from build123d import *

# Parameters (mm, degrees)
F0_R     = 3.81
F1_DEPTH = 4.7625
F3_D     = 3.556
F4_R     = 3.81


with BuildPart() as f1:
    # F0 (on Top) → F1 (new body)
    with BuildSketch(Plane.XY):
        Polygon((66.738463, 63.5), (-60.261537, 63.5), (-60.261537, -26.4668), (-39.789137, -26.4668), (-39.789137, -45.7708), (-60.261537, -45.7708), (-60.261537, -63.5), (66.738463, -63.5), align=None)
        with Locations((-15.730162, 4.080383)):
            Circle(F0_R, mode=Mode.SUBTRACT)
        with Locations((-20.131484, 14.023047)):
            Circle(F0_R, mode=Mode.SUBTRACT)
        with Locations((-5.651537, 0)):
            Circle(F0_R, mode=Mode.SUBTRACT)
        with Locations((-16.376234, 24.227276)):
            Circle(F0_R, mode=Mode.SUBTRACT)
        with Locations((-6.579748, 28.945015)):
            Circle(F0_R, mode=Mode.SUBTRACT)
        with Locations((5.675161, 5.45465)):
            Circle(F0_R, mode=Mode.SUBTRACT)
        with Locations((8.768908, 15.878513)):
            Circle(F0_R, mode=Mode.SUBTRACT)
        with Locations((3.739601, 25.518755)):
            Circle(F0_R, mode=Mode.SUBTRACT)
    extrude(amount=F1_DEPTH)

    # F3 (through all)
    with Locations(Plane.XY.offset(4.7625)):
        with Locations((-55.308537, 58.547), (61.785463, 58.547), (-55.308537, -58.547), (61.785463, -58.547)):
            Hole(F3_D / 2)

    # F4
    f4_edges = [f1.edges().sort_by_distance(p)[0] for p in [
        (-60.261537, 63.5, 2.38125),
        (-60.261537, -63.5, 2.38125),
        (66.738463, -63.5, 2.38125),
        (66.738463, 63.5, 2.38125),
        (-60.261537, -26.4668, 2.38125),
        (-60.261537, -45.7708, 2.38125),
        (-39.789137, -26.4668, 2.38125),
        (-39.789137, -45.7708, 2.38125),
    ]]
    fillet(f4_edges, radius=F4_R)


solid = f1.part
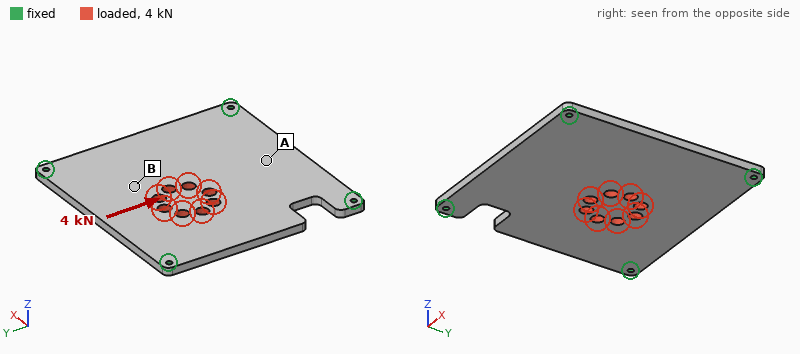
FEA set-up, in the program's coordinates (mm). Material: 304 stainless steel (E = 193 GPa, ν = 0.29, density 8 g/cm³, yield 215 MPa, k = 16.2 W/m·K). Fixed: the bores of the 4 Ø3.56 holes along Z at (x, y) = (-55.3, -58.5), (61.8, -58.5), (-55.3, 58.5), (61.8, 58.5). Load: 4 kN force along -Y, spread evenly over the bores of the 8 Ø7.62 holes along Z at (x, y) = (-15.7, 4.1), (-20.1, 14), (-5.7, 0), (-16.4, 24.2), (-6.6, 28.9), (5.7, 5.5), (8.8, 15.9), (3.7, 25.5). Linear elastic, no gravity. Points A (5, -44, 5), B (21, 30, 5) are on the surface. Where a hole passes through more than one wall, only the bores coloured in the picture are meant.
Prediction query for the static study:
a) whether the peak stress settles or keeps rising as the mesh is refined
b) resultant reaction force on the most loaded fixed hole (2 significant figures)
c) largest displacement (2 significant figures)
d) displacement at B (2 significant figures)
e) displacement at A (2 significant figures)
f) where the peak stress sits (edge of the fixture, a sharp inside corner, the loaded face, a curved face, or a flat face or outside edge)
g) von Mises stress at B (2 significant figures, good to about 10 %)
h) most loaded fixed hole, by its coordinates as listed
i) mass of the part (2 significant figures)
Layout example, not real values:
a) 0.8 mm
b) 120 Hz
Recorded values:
a) keeps rising
b) 1.6 kN
c) 6.3 µm
d) 4.0 µm
e) 3.9 µm
f) edge of the fixture
g) 8.6 MPa
h) (-55.3, 58.5)
i) 580 g
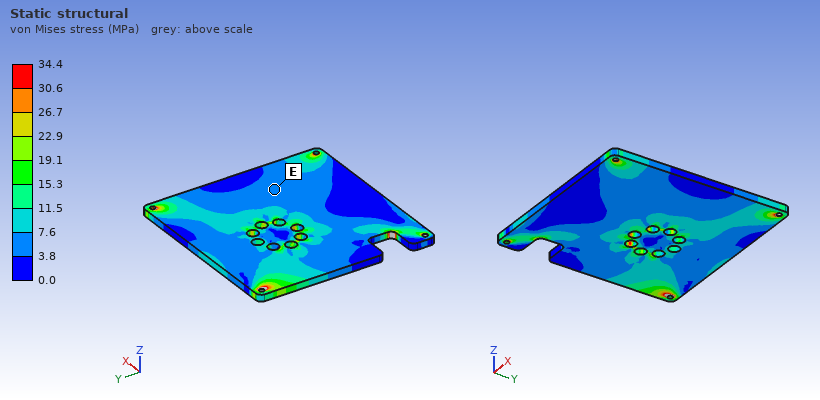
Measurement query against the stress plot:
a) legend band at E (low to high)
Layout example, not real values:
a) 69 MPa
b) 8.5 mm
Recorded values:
a) 3.8 to 7.6 MPa
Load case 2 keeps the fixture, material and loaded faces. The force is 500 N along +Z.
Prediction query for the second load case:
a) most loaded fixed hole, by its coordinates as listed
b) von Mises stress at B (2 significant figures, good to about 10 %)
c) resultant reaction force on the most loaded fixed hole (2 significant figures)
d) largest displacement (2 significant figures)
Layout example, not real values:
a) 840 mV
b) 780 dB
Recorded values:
a) (-55.3, 58.5)
b) 13 MPa
c) 200 N
d) 70 µm
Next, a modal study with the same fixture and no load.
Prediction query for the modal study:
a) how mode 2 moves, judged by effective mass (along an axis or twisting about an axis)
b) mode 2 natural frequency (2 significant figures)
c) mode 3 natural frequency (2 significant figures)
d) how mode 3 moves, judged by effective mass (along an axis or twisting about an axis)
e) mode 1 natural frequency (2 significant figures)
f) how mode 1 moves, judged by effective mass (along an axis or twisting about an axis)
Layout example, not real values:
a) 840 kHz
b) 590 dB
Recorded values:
a) twisting about Y
b) 1600 Hz
c) 1800 Hz
d) twisting about X
e) 950 Hz
f) along Z
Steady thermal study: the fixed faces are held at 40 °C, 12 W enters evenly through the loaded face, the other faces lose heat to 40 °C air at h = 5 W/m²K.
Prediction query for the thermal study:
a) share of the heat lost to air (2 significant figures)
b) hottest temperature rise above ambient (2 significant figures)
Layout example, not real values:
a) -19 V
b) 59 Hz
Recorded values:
a) 42 %
b) 69 K
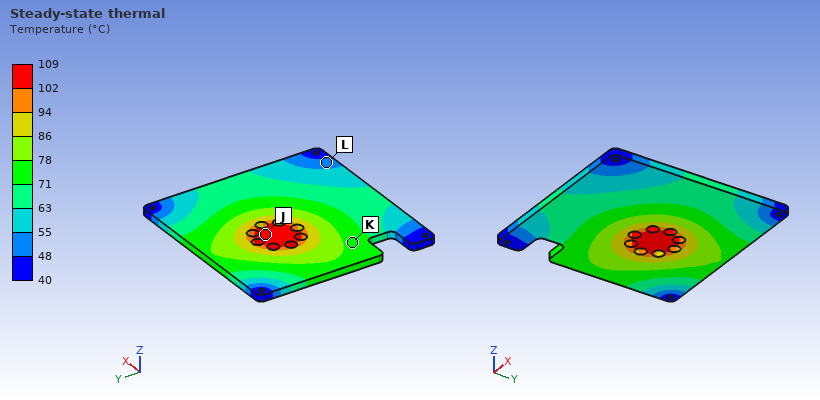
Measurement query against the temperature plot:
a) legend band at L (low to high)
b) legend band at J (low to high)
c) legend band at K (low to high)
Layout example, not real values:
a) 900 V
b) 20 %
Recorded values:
a) 48 to 55 °C
b) 102 to 109 °C
c) 71 to 78 °C
